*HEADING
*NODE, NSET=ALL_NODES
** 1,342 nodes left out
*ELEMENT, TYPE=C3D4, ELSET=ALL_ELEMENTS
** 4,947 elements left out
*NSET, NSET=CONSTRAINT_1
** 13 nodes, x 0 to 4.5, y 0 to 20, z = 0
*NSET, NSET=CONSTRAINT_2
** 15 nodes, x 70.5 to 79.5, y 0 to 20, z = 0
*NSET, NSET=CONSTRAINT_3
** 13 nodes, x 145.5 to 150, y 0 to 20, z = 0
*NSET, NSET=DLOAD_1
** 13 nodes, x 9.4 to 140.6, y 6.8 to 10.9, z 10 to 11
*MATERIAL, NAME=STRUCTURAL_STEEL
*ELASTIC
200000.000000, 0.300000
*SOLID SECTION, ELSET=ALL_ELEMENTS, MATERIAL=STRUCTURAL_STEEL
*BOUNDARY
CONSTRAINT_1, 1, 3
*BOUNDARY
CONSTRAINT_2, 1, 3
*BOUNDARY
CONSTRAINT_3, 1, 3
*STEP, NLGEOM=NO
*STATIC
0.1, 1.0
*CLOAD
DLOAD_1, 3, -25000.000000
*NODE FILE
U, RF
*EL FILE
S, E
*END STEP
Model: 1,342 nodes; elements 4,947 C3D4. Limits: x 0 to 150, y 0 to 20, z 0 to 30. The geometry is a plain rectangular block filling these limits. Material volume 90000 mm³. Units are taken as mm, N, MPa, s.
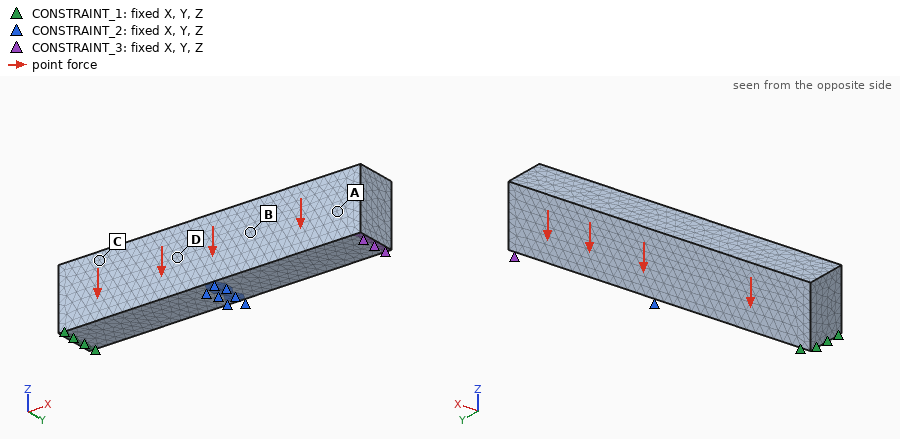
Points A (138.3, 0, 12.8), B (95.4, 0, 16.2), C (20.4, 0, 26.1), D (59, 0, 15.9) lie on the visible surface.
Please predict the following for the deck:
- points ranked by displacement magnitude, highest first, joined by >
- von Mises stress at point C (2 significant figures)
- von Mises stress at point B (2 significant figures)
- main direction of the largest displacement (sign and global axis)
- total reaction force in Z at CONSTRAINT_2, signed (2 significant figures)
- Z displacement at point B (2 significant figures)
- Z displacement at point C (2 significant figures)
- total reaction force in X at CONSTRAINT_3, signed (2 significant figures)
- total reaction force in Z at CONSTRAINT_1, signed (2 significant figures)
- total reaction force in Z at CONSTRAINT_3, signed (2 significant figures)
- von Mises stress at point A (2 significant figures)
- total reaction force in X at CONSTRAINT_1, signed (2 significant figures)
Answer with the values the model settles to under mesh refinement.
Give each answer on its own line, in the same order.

C > B > A > D
220 MPa
230 MPa
-Z
1.5e+05 N
-0.063 mm
-0.087 mm
-38000 N
96000 N
77000 N
280 MPa
38000 N
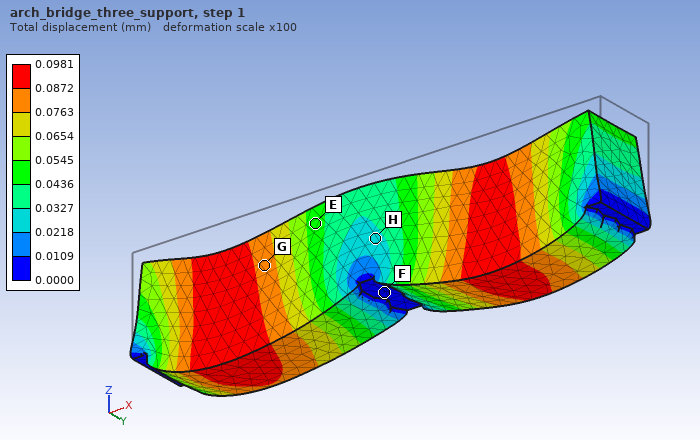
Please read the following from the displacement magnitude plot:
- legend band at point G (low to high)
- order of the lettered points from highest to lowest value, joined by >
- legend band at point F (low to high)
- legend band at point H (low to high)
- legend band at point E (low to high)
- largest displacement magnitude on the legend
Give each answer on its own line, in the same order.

0.0763 to 0.0872 mm
G > E > H > F
0.0000 to 0.0109 mm
0.0218 to 0.0327 mm
0.0436 to 0.0545 mm
0.0981 mm
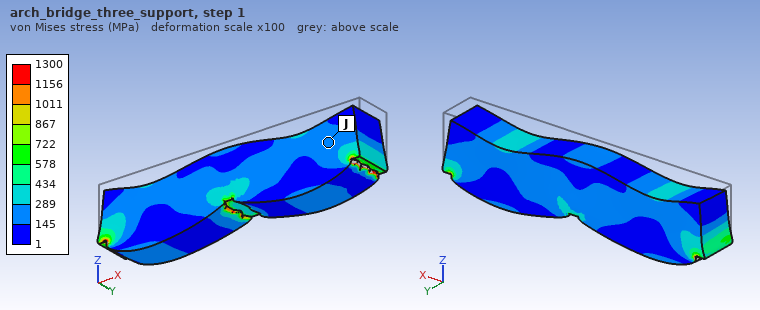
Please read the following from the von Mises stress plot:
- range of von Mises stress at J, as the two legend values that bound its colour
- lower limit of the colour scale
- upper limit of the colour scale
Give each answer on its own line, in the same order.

145 to 289 MPa
1 MPa
1300 MPa
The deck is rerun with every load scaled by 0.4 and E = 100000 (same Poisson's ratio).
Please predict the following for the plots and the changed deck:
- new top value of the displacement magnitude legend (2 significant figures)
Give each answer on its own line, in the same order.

0.078 mm
